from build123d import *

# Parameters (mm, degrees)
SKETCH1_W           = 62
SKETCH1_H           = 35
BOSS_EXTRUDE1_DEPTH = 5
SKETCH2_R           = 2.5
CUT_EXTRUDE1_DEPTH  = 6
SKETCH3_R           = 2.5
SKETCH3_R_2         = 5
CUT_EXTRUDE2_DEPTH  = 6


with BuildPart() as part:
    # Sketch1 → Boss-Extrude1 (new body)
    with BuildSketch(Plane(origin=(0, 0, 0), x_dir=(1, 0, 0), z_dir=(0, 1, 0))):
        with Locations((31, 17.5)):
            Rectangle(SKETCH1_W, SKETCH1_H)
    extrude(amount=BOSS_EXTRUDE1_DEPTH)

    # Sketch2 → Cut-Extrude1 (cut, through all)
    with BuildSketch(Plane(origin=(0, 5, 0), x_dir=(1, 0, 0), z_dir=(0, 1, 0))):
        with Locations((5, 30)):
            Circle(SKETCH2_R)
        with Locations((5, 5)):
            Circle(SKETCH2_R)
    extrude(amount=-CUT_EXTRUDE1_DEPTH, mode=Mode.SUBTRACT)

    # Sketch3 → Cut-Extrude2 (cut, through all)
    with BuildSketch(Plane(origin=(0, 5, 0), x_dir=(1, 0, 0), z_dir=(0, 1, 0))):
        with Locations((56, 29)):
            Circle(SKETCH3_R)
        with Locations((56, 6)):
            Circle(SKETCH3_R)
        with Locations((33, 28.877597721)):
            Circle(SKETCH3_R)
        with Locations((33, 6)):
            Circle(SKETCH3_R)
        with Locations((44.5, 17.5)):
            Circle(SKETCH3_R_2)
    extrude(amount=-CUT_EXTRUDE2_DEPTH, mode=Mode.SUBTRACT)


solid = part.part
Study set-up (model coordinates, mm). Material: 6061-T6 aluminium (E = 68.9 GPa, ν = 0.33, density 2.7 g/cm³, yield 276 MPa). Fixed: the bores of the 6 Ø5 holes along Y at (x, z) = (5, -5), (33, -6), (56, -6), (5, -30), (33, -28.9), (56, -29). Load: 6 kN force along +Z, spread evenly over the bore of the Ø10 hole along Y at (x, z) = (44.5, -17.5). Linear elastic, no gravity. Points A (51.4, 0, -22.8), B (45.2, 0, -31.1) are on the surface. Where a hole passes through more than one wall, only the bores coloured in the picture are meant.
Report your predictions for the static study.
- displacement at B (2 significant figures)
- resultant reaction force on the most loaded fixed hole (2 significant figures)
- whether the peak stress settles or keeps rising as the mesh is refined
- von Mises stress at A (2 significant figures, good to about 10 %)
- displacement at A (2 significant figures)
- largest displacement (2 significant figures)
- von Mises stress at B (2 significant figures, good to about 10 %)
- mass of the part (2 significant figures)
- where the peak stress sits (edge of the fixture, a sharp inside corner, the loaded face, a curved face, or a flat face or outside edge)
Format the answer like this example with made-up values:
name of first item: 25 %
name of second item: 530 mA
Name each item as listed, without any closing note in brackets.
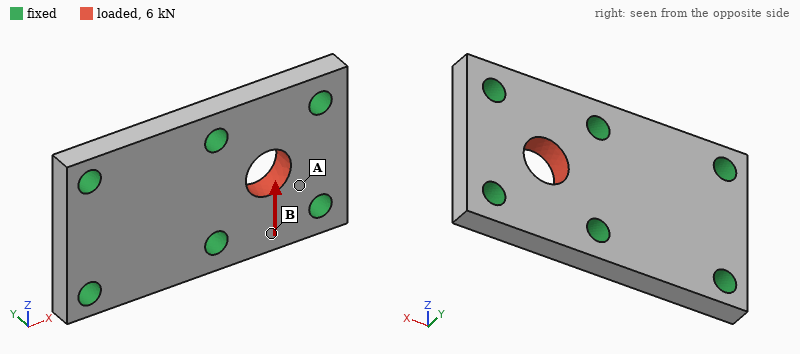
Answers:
displacement at B: 5.1 µm
resultant reaction force on the most loaded fixed hole: 1.6 kN
whether the peak stress settles or keeps rising as the mesh is refined: keeps rising
von Mises stress at A: 35 MPa
displacement at A: 3.4 µm
largest displacement: 7.8 µm
von Mises stress at B: 11 MPa
mass of the part: 27 g
where the peak stress sits: edge of the fixture
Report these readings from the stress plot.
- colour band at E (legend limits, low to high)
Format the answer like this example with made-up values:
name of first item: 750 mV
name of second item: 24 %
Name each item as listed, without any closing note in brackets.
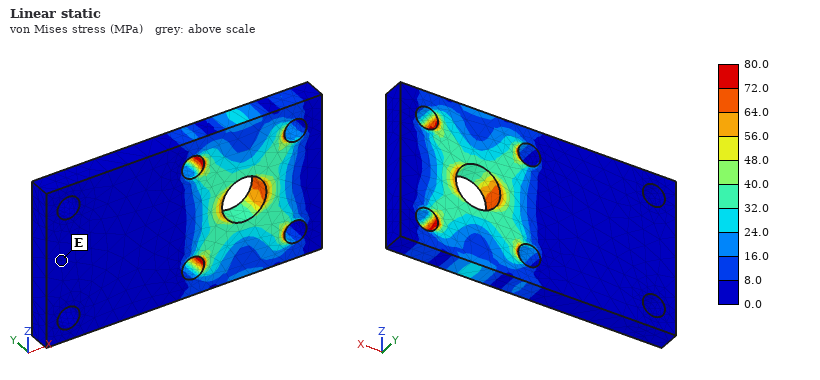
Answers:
colour band at E: 0.0 to 8.0 MPa
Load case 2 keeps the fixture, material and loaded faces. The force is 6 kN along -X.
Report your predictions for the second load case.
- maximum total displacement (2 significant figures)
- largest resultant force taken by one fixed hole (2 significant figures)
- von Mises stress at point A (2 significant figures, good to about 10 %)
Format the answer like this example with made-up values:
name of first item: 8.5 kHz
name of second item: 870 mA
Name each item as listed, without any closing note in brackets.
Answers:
maximum total displacement: 7.9 µm
largest resultant force taken by one fixed hole: 1.5 kN
von Mises stress at point A: 35 MPa
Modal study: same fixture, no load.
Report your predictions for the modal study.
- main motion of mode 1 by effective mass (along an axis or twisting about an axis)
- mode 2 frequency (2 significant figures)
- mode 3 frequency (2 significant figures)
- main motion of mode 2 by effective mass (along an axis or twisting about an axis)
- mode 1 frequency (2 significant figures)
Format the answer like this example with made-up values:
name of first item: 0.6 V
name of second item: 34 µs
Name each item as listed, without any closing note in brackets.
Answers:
main motion of mode 1 by effective mass: along Y
mode 2 frequency: 36 kHz
mode 3 frequency: 39 kHz
main motion of mode 2 by effective mass: twisting about X
mode 1 frequency: 27 kHz
